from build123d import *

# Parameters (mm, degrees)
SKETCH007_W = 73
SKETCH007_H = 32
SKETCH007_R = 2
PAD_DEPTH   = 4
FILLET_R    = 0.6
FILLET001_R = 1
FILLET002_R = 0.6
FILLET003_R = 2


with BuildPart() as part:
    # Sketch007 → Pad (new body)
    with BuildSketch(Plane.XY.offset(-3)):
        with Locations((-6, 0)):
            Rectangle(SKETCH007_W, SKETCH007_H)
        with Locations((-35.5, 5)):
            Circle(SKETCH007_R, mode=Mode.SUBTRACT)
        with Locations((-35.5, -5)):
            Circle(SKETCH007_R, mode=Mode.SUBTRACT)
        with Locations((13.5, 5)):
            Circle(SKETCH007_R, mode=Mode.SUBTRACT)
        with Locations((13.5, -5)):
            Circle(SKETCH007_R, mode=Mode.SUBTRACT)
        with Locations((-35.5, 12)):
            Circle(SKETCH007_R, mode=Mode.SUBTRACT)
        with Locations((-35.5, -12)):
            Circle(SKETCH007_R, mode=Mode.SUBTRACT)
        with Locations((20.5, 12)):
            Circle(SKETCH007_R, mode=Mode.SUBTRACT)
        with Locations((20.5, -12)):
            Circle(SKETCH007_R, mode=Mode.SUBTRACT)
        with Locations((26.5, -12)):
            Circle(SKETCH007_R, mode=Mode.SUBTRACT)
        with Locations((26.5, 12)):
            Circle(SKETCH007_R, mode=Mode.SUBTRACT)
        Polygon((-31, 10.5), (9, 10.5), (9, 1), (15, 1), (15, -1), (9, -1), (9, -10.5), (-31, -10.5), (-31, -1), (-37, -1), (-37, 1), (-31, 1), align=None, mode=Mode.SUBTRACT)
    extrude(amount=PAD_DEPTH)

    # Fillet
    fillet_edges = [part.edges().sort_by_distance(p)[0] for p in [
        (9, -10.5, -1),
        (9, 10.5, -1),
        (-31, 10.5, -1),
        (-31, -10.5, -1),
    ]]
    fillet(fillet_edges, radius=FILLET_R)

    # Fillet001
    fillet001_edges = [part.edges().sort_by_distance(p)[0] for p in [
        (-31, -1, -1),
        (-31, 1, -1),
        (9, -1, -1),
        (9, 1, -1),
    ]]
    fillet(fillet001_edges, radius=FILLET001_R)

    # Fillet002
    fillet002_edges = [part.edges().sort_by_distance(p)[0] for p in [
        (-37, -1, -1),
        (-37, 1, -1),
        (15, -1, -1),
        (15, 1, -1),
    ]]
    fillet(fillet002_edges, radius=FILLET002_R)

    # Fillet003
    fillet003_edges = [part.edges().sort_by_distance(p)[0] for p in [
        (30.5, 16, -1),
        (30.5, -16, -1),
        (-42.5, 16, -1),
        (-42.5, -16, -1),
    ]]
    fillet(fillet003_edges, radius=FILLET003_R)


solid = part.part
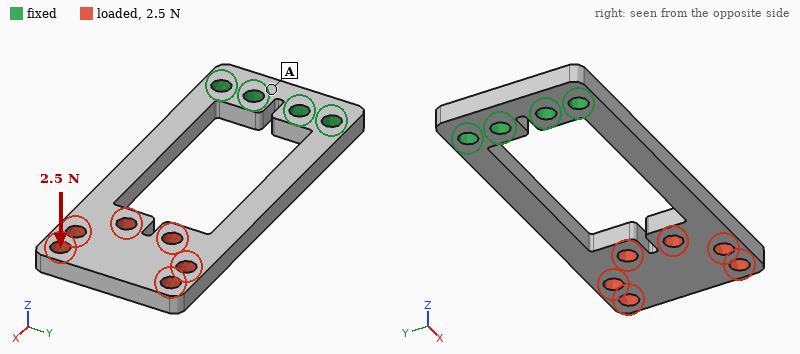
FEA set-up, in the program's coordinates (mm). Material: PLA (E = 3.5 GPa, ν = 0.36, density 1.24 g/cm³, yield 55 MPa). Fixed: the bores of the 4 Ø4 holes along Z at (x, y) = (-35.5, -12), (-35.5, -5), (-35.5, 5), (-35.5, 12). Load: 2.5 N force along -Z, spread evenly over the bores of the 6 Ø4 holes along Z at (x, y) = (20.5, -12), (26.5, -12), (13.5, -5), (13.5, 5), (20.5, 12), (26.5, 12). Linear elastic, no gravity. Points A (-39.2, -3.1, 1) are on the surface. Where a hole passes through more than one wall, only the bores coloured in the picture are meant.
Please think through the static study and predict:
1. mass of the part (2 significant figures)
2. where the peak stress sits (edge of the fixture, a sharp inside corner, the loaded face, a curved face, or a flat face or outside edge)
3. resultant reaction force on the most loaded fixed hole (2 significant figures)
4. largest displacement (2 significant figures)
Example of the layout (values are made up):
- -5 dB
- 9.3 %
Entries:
- 6.7 g
- a curved face
- 1.6 N
- 0.81 mm
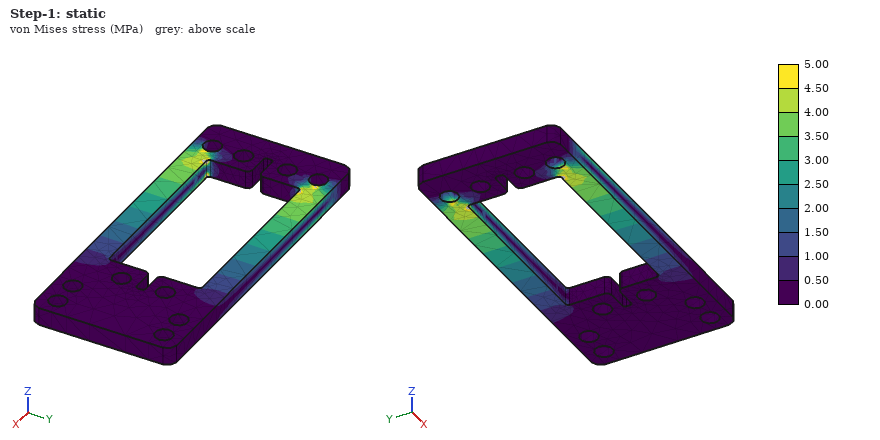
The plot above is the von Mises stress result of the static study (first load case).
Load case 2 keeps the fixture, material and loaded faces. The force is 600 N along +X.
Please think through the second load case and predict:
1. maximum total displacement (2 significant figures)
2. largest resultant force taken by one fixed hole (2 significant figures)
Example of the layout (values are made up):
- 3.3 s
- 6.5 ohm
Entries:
- 0.26 mm
- 310 N
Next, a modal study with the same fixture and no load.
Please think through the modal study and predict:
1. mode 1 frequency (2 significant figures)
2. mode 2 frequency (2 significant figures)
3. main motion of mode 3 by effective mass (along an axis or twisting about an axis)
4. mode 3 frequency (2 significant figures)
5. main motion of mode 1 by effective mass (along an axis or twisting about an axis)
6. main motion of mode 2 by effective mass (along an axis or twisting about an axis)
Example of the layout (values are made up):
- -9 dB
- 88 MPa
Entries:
- 180 Hz
- 550 Hz
- twisting about X
- 680 Hz
- along Z
- along Y
